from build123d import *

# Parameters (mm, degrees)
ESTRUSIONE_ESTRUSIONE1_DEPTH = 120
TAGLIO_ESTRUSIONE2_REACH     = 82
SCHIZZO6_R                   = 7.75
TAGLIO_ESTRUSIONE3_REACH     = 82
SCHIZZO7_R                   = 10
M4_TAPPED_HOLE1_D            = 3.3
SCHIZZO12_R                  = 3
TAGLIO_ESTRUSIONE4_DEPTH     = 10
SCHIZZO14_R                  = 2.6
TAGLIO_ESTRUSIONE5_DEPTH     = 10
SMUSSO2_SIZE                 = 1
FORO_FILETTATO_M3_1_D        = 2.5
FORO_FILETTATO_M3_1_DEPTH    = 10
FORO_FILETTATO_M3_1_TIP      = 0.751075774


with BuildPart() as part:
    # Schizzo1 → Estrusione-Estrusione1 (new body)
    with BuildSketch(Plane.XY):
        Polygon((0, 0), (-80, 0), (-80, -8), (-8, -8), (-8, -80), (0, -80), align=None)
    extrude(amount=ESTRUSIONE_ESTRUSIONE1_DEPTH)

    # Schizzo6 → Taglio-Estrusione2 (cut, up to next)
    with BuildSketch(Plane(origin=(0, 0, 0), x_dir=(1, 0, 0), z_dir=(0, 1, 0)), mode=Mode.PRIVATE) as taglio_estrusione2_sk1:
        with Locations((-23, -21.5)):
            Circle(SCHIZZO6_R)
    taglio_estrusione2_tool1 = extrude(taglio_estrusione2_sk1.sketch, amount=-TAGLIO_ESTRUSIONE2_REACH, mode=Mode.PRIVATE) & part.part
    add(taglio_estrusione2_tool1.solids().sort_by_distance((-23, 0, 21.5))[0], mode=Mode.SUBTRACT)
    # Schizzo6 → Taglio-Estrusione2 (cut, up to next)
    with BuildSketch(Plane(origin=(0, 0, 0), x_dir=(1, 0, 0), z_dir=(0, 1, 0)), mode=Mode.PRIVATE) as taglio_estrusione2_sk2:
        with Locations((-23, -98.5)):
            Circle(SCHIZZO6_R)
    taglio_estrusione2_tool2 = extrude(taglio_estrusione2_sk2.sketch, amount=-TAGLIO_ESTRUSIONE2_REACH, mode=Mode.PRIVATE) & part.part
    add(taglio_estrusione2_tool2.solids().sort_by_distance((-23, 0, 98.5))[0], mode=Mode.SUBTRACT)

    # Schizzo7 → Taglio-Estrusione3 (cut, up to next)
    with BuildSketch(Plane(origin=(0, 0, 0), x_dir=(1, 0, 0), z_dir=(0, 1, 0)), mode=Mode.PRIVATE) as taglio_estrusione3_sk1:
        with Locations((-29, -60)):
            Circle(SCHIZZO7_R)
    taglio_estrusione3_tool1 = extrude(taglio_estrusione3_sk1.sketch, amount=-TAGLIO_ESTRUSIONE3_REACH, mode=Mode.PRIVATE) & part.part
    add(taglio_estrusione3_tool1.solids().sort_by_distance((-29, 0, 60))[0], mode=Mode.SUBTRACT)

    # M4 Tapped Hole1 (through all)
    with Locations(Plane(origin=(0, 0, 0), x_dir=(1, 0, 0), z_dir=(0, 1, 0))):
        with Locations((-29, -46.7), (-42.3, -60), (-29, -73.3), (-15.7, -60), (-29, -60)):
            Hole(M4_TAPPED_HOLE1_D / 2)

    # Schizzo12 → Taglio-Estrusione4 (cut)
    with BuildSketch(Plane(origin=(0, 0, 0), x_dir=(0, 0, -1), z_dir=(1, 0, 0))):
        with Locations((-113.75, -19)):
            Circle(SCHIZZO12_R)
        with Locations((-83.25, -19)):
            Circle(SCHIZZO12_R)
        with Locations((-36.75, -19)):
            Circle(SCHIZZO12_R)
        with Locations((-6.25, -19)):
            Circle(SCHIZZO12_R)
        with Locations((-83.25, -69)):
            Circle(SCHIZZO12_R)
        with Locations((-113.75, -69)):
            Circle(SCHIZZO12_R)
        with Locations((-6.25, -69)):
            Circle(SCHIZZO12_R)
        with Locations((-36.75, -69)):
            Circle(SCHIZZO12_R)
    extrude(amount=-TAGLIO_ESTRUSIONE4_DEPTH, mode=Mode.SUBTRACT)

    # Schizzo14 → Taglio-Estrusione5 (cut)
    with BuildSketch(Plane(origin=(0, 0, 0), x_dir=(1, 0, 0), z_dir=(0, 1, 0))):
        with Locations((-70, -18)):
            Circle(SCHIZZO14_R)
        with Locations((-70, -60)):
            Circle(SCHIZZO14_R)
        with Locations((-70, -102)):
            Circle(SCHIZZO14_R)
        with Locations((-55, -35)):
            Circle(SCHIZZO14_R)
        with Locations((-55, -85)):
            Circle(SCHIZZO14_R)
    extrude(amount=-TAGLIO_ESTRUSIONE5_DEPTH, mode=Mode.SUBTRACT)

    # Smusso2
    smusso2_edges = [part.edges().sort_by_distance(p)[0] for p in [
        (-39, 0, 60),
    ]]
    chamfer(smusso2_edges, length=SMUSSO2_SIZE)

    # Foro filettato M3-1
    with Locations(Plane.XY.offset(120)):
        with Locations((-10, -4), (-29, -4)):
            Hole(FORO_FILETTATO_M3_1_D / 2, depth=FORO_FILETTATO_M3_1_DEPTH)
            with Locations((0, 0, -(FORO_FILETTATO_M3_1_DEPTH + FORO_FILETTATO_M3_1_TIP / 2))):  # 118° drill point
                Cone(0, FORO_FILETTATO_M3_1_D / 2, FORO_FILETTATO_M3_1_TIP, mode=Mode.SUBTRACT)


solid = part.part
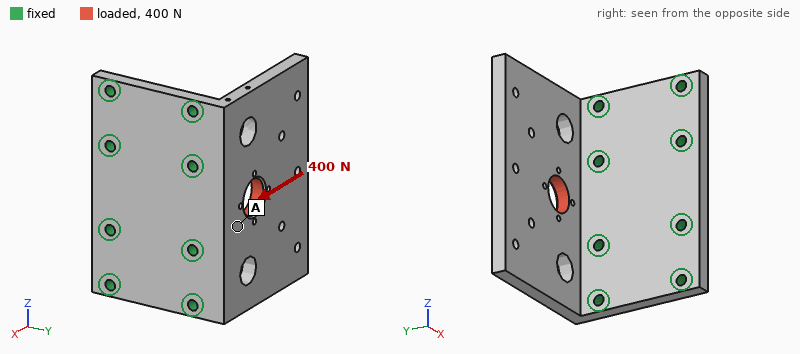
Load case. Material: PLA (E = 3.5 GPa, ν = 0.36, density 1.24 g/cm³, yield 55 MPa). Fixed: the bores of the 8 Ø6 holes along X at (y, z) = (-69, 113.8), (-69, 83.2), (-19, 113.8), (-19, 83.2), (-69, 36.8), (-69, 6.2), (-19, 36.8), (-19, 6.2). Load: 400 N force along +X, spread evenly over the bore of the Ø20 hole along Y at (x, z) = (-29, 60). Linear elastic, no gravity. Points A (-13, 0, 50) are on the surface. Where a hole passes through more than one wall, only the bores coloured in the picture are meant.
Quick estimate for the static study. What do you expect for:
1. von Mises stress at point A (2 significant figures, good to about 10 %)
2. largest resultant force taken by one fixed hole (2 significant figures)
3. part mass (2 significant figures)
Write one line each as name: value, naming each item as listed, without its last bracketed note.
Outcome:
von Mises stress at point A: 0.68 MPa
largest resultant force taken by one fixed hole: 140 N
part mass: 170 g
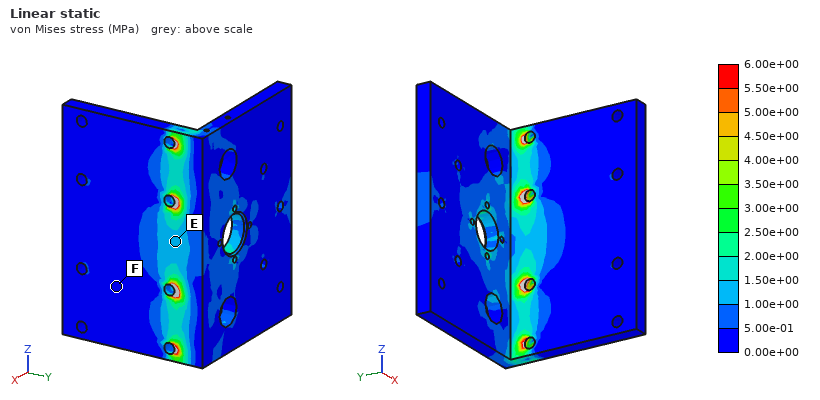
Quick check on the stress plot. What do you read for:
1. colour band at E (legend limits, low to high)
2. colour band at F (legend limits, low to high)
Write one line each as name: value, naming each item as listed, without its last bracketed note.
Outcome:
colour band at E: 1.00e+00 to 1.50e+00 MPa
colour band at F: 0.00e+00 to 5.00e-01 MPa
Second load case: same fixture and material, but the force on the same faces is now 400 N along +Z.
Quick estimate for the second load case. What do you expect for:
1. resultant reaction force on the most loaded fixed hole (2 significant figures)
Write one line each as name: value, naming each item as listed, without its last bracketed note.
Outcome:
resultant reaction force on the most loaded fixed hole: 130 N
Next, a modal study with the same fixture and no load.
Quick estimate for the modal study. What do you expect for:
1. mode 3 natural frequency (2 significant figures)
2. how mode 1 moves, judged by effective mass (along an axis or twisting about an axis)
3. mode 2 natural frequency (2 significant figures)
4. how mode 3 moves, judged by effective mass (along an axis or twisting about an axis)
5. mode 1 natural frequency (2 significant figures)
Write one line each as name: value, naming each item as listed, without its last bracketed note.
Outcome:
mode 3 natural frequency: 1300 Hz
how mode 1 moves, judged by effective mass: along Y
mode 2 natural frequency: 540 Hz
how mode 3 moves, judged by effective mass: along Z
mode 1 natural frequency: 280 Hz
